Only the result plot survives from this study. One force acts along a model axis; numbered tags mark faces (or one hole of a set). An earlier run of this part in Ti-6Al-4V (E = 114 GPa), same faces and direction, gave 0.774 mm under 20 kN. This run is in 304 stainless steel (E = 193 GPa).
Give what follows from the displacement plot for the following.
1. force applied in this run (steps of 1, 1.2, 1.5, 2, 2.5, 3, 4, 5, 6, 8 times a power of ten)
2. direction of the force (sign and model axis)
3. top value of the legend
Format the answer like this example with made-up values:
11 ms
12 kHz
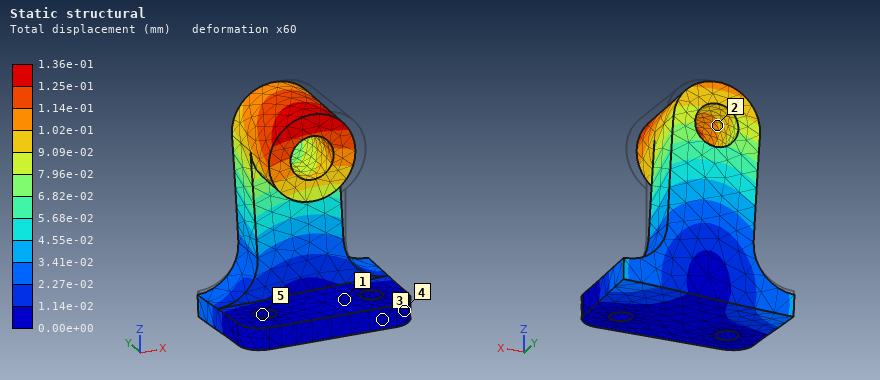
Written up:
6 kN
-X
1.36e-01 mm
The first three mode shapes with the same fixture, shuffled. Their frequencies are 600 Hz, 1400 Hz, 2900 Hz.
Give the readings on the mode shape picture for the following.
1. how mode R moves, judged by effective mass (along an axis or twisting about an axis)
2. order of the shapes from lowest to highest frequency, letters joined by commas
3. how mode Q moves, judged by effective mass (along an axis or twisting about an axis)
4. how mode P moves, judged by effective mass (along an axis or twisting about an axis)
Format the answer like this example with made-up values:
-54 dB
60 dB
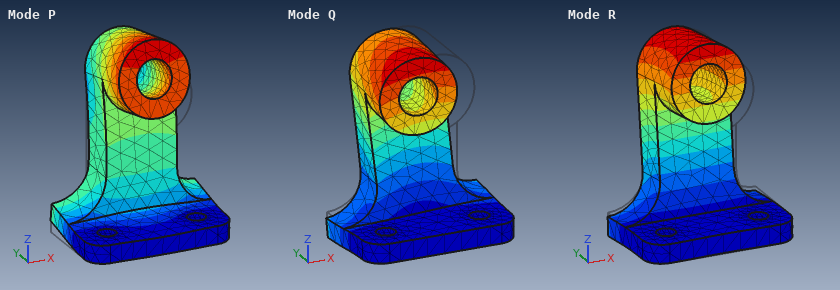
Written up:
along Y
R, Q, P
along X
along Z
